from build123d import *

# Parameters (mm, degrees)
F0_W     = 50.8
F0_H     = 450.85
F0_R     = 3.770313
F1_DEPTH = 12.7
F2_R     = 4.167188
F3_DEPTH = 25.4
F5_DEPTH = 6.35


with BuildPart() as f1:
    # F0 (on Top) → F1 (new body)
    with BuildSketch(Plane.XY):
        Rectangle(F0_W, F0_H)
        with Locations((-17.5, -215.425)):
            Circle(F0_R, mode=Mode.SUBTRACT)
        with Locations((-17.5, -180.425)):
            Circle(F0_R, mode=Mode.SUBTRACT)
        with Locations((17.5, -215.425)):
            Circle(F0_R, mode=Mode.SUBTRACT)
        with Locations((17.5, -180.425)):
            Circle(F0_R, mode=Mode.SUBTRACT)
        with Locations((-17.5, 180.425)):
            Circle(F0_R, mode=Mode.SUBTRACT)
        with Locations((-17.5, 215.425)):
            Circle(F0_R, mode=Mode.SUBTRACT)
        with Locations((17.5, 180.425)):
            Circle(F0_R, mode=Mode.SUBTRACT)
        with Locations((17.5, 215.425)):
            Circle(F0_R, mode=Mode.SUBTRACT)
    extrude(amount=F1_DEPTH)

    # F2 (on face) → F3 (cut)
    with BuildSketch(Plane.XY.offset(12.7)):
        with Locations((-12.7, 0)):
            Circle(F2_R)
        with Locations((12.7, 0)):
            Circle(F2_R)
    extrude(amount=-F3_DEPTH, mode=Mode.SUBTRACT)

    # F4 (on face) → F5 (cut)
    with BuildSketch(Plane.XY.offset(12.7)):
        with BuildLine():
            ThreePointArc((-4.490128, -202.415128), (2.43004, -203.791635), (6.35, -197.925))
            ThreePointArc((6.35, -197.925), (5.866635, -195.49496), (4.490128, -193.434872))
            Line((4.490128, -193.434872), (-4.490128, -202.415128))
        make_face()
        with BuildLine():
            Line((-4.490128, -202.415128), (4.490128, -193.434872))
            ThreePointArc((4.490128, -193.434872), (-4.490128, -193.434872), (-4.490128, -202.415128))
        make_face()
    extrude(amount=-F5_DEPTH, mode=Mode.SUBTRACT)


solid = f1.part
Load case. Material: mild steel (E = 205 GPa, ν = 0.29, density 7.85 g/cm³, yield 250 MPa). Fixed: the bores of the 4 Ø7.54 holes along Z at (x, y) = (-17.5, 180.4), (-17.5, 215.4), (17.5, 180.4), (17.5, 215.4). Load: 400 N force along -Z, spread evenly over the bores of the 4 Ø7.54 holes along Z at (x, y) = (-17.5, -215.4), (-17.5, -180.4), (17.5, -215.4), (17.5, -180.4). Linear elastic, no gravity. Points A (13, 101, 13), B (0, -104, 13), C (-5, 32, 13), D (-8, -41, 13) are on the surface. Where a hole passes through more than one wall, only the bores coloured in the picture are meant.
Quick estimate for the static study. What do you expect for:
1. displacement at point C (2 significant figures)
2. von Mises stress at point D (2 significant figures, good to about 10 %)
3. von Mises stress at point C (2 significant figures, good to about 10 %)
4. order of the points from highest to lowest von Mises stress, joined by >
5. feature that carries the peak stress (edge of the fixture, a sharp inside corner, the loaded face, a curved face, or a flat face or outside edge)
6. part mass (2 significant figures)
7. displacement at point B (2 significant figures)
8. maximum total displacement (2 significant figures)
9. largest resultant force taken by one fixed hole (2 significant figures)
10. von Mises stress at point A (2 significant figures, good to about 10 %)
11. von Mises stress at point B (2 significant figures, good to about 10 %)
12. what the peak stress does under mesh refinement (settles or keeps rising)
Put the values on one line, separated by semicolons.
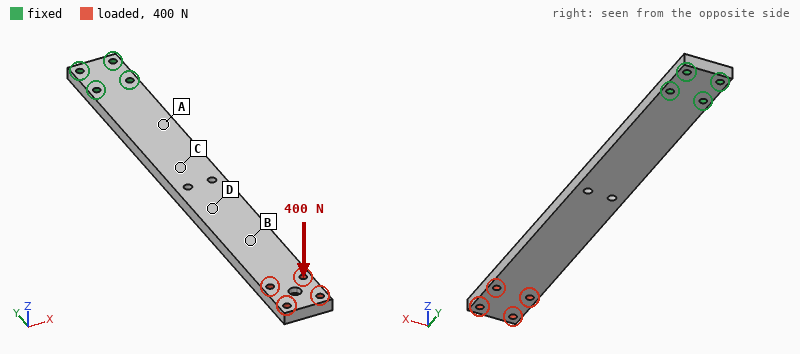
0.81 mm; 46 MPa; 68 MPa; A > C > D > B; edge of the fixture; 2.2 kg; 2.6 mm; 4.5 mm; 660 N; 88 MPa; 27 MPa; keeps rising
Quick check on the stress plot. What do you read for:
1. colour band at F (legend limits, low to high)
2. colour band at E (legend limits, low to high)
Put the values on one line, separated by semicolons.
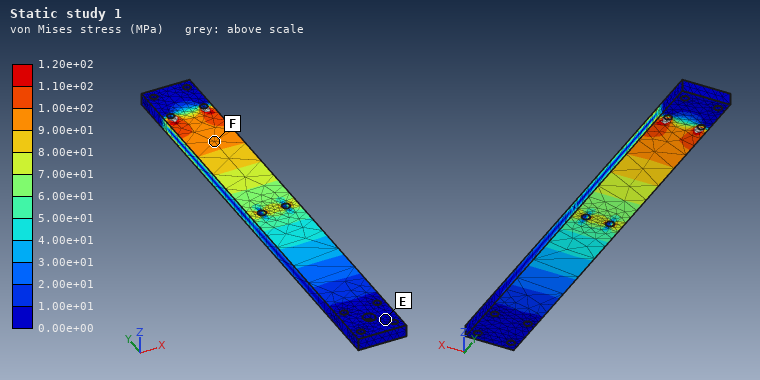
9.00e+01 to 1.00e+02 MPa; 0.00e+00 to 1.00e+01 MPa
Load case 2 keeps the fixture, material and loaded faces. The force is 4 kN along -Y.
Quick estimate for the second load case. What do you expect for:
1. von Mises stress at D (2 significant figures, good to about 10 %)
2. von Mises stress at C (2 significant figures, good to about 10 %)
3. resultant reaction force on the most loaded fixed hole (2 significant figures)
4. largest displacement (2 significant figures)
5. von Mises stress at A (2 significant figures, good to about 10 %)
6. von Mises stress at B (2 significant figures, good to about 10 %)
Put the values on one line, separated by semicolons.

6.2 MPa; 6.1 MPa; 1.8 kN; 12 µm; 6.2 MPa; 6.2 MPa
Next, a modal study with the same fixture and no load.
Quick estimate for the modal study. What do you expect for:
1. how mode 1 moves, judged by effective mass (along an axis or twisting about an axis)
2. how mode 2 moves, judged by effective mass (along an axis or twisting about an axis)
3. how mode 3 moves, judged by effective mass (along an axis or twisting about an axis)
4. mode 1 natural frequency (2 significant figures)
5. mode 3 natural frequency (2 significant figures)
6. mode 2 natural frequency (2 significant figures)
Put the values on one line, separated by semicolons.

along Z; along X; along Z; 65 Hz; 400 Hz; 260 Hz
